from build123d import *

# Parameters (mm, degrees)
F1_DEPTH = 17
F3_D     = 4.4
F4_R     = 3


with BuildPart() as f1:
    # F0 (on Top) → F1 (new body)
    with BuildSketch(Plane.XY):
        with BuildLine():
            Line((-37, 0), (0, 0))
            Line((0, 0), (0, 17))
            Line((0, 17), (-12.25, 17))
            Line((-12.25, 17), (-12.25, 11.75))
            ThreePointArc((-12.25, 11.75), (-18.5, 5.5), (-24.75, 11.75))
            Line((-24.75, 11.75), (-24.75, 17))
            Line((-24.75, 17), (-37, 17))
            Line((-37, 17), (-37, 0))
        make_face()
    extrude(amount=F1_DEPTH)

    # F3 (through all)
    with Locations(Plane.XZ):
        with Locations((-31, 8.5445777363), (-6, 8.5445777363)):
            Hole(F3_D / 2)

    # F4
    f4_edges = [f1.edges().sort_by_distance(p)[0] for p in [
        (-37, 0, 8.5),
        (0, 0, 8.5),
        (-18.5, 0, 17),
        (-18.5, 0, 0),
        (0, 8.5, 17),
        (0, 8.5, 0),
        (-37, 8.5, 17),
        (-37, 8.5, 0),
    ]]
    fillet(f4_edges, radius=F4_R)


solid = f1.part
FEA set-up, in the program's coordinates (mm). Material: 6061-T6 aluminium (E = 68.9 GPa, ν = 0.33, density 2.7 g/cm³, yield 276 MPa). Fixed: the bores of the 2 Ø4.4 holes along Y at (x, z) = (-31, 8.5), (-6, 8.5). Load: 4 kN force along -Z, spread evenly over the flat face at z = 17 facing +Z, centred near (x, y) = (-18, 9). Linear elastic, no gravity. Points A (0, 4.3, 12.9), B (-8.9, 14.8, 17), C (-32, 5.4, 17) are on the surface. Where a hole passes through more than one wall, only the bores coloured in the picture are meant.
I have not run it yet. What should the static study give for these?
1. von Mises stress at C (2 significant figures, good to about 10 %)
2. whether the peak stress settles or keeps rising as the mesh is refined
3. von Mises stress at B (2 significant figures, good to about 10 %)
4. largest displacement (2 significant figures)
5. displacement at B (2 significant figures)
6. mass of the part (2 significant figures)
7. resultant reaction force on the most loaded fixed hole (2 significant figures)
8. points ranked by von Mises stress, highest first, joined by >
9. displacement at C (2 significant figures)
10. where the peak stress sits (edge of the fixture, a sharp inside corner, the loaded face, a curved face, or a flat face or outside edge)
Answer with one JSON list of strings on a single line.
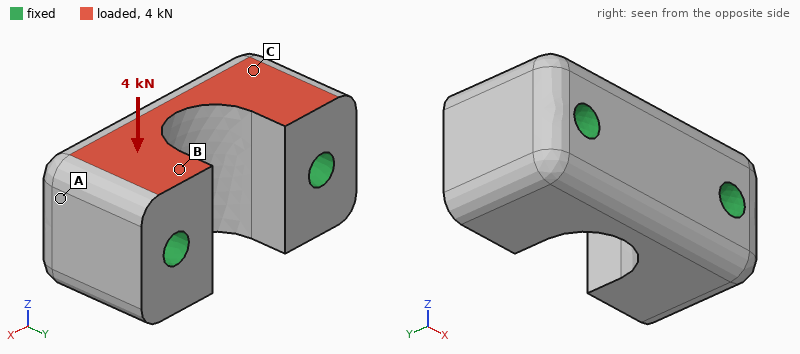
["8.5 MPa", "keeps rising", "14 MPa", "3.1 µm", "2.4 µm", "21 g", "2.0 kN", "B > C > A", "1.3 µm", "edge of the fixture"]
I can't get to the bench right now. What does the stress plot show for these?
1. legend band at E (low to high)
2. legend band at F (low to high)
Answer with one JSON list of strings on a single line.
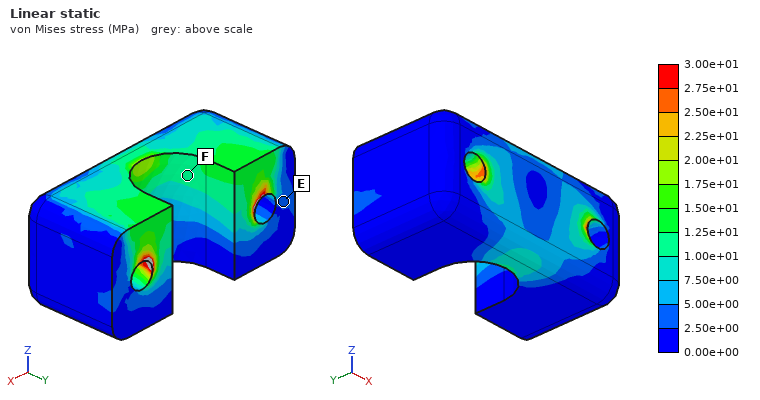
["2.50e+00 to 5.00e+00 MPa", "1.00e+01 to 1.25e+01 MPa"]
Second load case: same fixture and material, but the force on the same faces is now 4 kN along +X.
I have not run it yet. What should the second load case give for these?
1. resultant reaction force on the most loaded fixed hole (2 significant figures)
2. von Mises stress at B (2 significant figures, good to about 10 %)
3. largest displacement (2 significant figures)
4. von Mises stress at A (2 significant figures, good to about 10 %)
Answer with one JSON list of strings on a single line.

["2.1 kN", "27 MPa", "8.7 µm", "12 MPa"]
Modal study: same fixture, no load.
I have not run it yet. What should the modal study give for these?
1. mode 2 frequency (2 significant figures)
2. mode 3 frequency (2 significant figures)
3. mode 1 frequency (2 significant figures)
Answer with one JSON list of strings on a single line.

["61 kHz", "62 kHz", "48 kHz"]
